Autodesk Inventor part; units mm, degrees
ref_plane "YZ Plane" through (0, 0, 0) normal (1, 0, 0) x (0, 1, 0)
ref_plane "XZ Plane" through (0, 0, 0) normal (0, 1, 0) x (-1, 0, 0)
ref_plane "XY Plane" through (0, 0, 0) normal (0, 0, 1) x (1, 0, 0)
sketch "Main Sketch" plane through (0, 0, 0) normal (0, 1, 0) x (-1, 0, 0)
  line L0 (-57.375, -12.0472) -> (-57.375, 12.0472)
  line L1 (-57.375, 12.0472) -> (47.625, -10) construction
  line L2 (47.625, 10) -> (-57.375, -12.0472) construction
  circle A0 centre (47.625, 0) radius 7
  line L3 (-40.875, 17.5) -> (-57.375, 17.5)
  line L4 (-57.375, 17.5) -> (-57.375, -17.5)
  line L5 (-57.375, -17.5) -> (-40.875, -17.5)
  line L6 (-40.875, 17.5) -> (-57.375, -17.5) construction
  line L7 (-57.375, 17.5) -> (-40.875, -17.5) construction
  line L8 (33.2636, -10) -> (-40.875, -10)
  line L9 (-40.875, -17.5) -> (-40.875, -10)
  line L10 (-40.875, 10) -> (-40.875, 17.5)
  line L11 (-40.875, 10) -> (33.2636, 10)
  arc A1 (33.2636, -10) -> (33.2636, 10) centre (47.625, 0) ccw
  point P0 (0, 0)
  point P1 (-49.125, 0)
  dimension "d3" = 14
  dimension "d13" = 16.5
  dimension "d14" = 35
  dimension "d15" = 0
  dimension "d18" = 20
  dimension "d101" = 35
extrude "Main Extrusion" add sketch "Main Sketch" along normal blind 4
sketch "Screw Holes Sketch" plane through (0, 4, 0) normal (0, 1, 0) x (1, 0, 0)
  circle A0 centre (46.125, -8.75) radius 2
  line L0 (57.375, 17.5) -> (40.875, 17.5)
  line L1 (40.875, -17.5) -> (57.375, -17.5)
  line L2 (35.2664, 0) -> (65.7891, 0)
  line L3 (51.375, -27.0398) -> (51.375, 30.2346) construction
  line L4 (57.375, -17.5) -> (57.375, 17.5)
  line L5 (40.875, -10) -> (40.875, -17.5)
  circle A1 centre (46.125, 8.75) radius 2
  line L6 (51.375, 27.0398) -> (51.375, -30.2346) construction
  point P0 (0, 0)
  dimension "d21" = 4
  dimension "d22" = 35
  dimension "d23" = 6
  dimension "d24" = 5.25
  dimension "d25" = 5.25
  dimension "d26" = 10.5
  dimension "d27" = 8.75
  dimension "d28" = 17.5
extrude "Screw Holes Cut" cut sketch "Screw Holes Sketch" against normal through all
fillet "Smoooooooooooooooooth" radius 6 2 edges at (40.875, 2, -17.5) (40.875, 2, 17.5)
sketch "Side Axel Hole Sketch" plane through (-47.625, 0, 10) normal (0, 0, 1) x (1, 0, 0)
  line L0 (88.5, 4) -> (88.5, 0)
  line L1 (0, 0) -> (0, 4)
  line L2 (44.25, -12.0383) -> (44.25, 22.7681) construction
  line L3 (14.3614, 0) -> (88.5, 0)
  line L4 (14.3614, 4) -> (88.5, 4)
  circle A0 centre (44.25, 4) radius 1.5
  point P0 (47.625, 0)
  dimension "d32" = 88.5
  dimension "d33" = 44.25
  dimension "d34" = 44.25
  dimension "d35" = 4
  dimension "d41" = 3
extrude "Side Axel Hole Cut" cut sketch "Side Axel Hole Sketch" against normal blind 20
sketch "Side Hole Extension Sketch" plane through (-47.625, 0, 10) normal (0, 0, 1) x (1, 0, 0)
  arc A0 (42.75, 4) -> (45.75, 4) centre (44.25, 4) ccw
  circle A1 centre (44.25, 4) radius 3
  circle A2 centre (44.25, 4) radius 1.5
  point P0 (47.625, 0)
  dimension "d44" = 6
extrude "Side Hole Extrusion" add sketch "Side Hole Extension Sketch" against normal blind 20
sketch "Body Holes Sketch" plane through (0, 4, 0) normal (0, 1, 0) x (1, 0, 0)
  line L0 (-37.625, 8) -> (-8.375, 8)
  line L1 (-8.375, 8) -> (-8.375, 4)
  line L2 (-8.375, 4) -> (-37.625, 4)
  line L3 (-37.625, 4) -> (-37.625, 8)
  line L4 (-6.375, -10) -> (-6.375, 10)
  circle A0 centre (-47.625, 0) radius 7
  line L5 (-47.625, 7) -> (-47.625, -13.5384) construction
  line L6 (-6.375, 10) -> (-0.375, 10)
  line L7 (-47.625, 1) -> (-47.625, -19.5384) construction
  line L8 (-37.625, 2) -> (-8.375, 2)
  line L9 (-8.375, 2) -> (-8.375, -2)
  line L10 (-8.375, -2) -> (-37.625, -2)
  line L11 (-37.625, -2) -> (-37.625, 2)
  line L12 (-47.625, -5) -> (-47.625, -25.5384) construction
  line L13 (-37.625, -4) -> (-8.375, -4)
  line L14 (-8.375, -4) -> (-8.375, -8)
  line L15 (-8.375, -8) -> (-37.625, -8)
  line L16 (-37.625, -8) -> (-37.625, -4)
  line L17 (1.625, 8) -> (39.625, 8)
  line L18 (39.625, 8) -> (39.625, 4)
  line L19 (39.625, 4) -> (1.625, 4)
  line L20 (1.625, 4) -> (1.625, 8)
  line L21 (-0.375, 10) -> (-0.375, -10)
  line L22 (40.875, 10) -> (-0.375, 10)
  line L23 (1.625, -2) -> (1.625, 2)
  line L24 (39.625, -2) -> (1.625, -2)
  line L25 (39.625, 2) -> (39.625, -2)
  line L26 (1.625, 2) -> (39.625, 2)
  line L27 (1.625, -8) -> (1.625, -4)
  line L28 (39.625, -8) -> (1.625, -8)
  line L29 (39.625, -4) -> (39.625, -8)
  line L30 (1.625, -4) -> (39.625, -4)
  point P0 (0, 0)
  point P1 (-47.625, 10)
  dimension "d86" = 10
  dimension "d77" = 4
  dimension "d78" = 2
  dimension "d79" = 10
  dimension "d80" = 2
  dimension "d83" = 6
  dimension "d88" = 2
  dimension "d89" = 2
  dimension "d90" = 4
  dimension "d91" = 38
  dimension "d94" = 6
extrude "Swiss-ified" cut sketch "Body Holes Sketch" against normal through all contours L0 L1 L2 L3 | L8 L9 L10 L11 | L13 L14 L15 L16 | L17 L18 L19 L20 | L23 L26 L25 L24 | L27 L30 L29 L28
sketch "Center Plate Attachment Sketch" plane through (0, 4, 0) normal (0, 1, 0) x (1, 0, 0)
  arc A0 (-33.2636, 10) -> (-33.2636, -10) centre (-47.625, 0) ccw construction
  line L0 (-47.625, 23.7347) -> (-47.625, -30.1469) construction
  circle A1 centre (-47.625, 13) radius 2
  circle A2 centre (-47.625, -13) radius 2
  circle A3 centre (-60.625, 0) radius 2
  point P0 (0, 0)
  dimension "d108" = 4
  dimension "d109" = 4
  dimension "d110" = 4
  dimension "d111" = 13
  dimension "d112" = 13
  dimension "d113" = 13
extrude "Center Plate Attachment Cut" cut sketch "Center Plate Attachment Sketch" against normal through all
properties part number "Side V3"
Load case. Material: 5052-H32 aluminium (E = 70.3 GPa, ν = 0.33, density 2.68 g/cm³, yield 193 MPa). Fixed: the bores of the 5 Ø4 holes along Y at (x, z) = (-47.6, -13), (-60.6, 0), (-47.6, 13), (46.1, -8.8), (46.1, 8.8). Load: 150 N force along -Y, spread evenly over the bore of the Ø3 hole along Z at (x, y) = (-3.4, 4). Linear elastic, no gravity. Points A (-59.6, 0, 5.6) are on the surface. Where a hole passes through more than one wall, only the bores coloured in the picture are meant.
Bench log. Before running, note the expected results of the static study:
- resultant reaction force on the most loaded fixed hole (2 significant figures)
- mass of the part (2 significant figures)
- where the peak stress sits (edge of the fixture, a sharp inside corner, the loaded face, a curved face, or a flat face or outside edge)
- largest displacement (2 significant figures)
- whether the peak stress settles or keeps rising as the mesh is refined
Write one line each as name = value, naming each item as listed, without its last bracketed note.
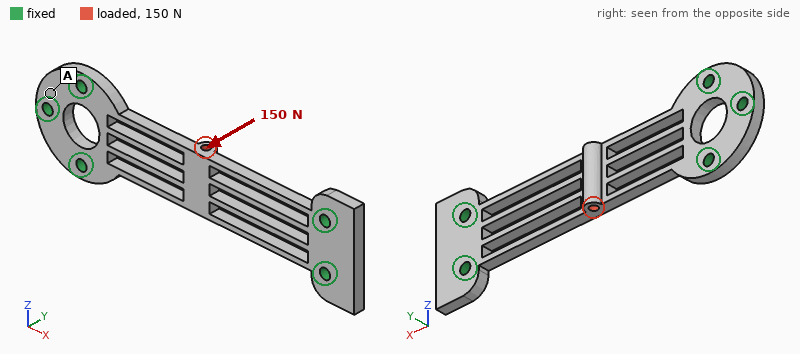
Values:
resultant reaction force on the most loaded fixed hole = 50 N
mass of the part = 21 g
where the peak stress sits = a sharp inside corner
largest displacement = 0.14 mm
whether the peak stress settles or keeps rising as the mesh is refined = keeps rising
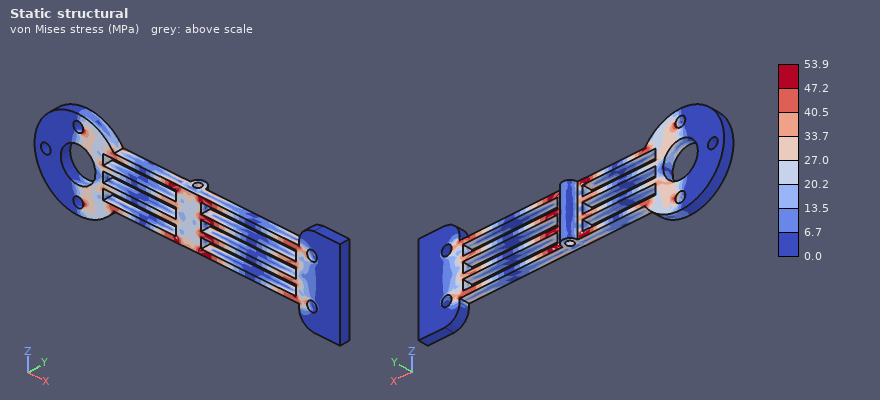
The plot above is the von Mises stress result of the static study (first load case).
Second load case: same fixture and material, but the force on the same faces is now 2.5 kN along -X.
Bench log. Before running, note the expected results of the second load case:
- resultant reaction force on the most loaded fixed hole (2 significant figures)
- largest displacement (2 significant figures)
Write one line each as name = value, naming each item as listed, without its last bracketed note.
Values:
resultant reaction force on the most loaded fixed hole = 680 N
largest displacement = 84 µm
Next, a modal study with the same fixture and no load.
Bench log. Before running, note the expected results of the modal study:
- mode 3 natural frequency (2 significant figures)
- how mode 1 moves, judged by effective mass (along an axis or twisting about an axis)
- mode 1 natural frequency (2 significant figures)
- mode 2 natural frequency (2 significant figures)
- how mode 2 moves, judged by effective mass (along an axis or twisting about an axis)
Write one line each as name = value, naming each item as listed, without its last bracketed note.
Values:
mode 3 natural frequency = 3800 Hz
how mode 1 moves, judged by effective mass = along Z
mode 1 natural frequency = 1700 Hz
mode 2 natural frequency = 2400 Hz
how mode 2 moves, judged by effective mass = along Y
